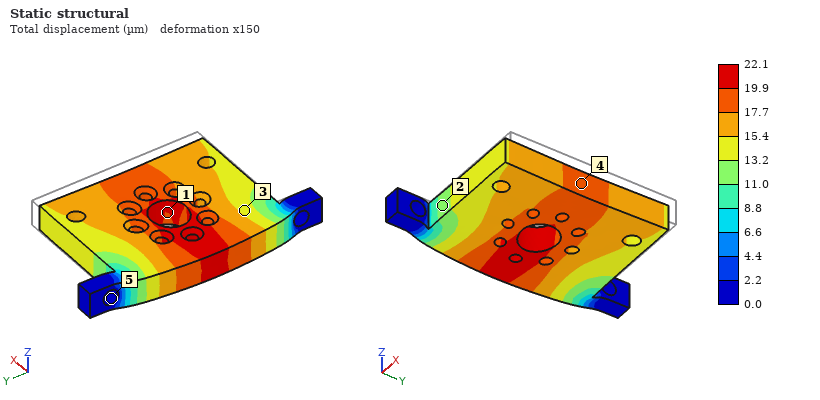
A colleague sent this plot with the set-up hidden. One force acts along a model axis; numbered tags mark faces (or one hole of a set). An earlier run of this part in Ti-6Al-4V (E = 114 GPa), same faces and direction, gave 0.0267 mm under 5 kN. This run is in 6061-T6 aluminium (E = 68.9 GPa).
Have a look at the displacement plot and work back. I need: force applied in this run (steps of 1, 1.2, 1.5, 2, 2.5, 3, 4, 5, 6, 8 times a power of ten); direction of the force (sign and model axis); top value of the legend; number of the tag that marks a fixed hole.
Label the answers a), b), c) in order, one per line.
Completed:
a) 2.5 kN
b) -X
c) 22.1 µm
d) 5
